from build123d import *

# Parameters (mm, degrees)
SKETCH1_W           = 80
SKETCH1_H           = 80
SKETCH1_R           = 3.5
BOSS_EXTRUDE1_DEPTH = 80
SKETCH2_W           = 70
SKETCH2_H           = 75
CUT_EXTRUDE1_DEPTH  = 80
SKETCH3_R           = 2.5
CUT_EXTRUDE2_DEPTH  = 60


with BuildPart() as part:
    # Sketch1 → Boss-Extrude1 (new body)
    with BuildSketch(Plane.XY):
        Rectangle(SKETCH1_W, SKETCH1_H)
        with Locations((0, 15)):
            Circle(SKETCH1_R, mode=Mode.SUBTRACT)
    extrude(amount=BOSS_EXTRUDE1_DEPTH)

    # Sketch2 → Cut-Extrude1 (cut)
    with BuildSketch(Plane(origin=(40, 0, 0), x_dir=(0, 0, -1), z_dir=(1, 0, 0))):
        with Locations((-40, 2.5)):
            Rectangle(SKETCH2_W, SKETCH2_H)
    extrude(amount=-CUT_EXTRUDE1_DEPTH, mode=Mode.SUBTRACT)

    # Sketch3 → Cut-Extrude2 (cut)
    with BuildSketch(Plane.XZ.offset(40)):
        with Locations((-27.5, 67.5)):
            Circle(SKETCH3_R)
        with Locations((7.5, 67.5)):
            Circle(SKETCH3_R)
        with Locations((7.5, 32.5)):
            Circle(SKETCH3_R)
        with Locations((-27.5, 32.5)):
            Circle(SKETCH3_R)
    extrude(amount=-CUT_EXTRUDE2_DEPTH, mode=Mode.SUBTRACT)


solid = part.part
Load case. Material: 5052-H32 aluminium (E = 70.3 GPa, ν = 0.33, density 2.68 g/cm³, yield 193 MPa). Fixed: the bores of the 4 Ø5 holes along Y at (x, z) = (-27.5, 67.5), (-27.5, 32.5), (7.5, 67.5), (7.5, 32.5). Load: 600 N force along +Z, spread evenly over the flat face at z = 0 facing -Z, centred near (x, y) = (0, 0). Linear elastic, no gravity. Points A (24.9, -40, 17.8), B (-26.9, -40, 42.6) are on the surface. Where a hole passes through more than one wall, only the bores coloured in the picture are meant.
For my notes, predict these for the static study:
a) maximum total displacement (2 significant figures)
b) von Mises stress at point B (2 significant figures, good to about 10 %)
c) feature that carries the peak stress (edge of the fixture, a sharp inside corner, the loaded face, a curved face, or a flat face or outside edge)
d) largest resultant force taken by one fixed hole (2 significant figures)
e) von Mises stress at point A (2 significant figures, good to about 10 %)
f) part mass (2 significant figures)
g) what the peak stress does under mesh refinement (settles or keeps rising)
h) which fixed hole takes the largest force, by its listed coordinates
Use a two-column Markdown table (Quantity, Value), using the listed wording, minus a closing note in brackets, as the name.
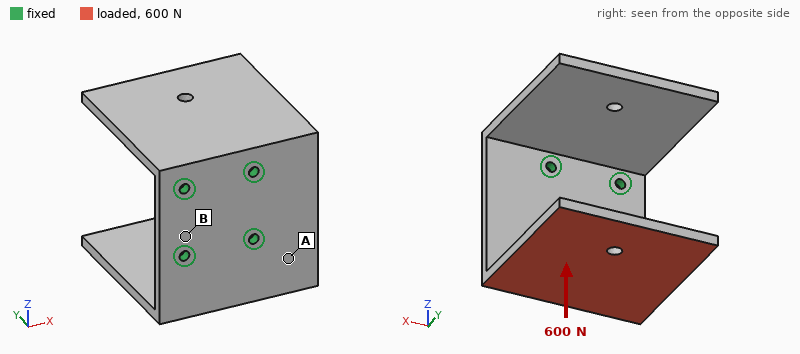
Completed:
| Quantity | Value |
|---|---|
| maximum total displacement | 1.4 mm |
| von Mises stress at point B | 9.6 MPa |
| feature that carries the peak stress | edge of the fixture |
| largest resultant force taken by one fixed hole | 400 N |
| von Mises stress at point A | 54 MPa |
| part mass | 240 g |
| what the peak stress does under mesh refinement | keeps rising |
| which fixed hole takes the largest force, by its listed coordinates | (7.5, 32.5) |
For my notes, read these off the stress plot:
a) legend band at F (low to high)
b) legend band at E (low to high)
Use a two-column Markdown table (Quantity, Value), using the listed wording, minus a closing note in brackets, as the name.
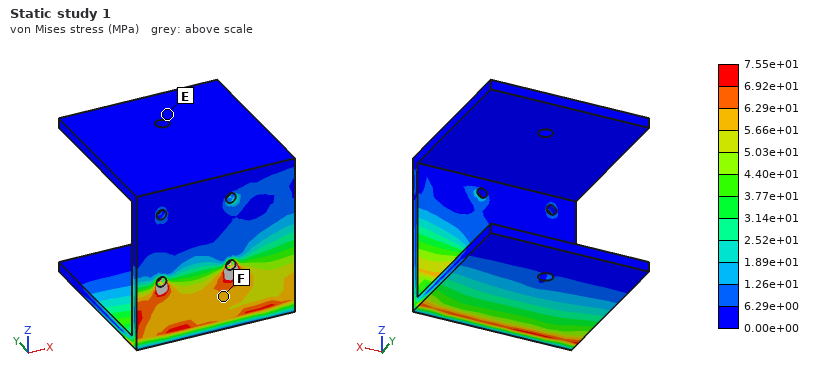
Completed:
| Quantity | Value |
|---|---|
| legend band at F | 5.66e+01 to 6.29e+01 MPa |
| legend band at E | 0.00e+00 to 6.29e+00 MPa |
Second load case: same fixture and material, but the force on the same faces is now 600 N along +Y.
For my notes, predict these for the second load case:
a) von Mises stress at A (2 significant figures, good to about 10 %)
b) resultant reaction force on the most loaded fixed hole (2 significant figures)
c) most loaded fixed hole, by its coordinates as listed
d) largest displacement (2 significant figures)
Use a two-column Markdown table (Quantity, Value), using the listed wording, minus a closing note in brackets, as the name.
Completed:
| Quantity | Value |
|---|---|
| von Mises stress at A | 25 MPa |
| resultant reaction force on the most loaded fixed hole | 570 N |
| most loaded fixed hole, by its coordinates as listed | (7.5, 32.5) |
| largest displacement | 0.51 mm |
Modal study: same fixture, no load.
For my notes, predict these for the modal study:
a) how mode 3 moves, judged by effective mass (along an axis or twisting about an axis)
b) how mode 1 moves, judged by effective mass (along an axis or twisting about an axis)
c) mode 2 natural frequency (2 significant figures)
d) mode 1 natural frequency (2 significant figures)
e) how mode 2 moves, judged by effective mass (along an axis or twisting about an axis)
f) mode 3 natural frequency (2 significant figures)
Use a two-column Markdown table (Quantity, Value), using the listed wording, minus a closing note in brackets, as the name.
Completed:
| Quantity | Value |
|---|---|
| how mode 3 moves, judged by effective mass | along X |
| how mode 1 moves, judged by effective mass | along Z |
| mode 2 natural frequency | 580 Hz |
| mode 1 natural frequency | 430 Hz |
| how mode 2 moves, judged by effective mass | along Z |
| mode 3 natural frequency | 870 Hz |
